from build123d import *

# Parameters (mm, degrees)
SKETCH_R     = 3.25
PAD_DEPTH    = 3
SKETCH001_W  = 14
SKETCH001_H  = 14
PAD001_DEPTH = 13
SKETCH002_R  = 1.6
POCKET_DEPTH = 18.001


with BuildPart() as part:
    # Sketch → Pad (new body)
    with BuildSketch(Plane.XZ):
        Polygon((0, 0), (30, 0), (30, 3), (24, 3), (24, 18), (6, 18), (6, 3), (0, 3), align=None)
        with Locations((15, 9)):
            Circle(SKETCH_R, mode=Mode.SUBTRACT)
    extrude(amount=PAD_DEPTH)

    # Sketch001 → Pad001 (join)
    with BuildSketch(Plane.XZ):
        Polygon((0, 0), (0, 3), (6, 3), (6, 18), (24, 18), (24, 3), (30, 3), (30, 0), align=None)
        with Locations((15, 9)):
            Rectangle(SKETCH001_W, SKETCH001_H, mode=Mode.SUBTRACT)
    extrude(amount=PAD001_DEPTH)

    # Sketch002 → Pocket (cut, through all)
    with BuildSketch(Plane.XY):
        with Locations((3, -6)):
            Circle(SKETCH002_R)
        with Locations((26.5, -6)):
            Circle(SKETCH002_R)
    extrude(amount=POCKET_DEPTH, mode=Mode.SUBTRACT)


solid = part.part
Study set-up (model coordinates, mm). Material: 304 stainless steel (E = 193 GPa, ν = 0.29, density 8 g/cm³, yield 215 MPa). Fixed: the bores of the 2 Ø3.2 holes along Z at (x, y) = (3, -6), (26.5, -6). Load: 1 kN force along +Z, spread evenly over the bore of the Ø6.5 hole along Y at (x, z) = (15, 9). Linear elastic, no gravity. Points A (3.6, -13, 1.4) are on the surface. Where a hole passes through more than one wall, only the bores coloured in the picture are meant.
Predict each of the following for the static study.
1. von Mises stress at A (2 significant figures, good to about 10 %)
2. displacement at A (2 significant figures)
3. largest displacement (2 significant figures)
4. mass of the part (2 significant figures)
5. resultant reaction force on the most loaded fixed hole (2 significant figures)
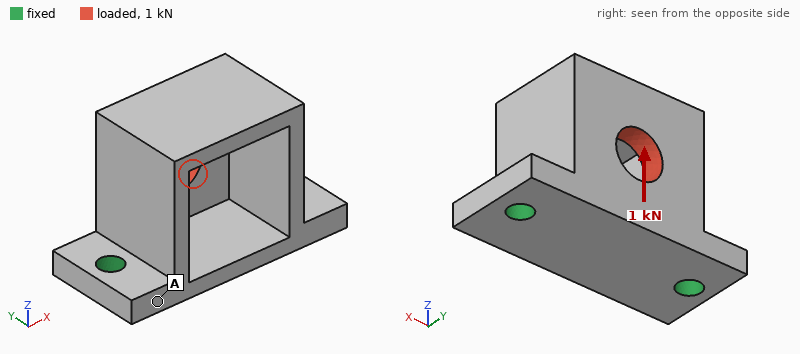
22 MPa
2.6 µm
17 µm
21 g
530 N
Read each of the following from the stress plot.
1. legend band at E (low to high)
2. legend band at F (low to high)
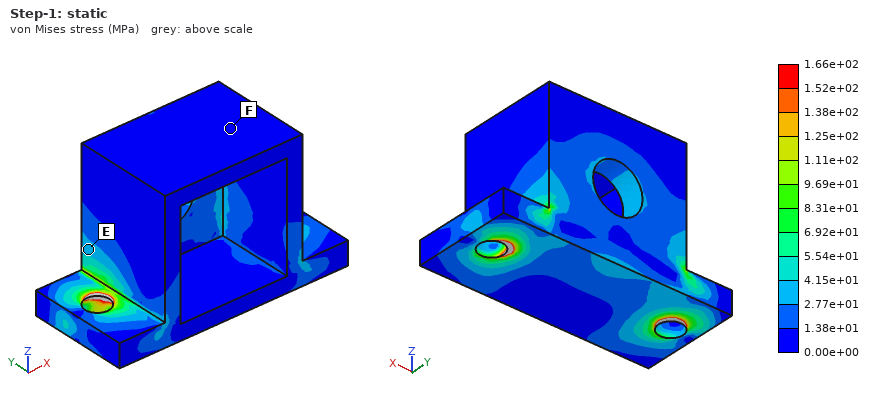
2.77e+01 to 4.15e+01 MPa
0.00e+00 to 1.38e+01 MPa
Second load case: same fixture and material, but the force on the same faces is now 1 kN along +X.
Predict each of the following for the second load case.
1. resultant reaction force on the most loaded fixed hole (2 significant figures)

650 N
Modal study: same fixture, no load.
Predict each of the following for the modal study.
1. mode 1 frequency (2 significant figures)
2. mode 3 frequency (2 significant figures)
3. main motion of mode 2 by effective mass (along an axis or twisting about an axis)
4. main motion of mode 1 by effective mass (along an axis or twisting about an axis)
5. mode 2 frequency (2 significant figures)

7800 Hz
23 kHz
along X
along Y
10 kHz
